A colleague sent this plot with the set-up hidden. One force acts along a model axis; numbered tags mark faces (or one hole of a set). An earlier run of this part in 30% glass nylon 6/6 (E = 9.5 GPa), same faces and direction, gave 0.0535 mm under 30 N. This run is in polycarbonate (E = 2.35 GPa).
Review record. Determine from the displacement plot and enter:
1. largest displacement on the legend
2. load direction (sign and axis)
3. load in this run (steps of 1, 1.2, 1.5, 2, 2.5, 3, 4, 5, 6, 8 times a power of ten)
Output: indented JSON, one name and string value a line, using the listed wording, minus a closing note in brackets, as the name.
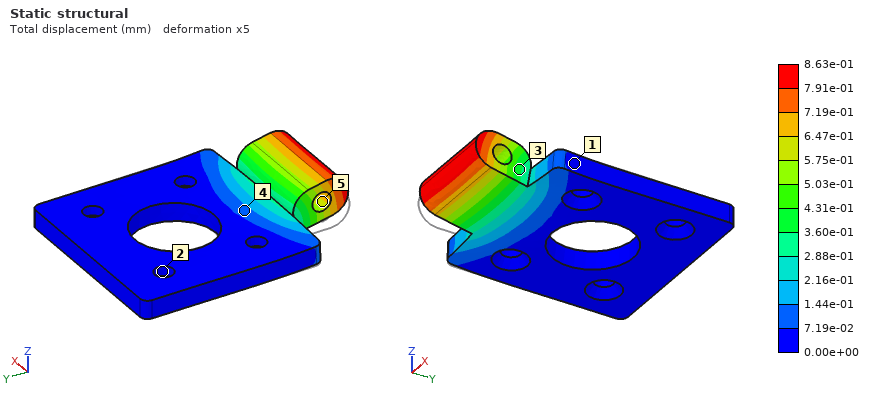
{
  "largest displacement on the legend": "8.63e-01 mm",
  "load direction": "+Z",
  "load in this run": "120 N"
}
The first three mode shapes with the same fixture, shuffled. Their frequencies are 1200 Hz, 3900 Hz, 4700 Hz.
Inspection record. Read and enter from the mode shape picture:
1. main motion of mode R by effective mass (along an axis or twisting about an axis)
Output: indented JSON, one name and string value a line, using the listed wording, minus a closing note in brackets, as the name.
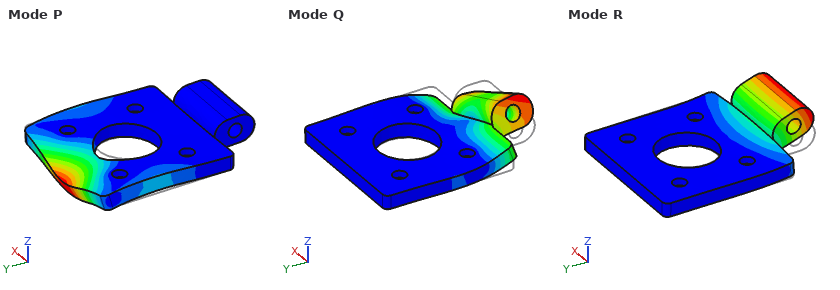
{
  "main motion of mode R by effective mass": "along Z"
}
